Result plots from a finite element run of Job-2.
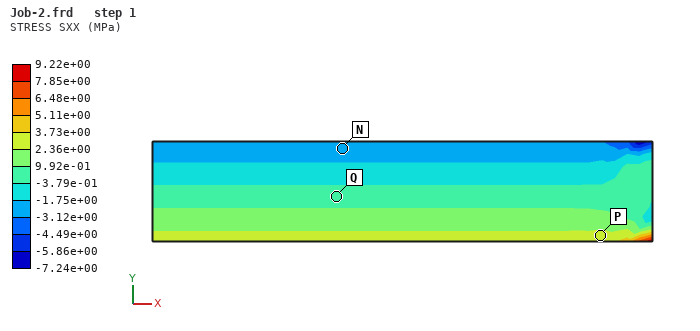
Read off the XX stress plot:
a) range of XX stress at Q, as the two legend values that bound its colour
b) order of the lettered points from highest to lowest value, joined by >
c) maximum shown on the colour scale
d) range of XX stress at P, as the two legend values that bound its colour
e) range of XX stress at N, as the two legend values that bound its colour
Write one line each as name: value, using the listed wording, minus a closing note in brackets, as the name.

range of XX stress at Q, as the two legend values that bound its colour: -3.79e-01 to 9.92e-01 MPa
order of the lettered points from highest to lowest value, joined by >: P > Q > N
maximum shown on the colour scale: 9.22e+00 MPa
range of XX stress at P, as the two legend values that bound its colour: 2.36e+00 to 3.73e+00 MPa
range of XX stress at N, as the two legend values that bound its colour: -3.12e+00 to -1.75e+00 MPa
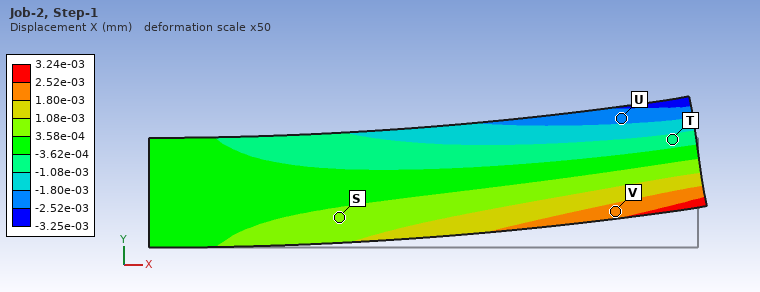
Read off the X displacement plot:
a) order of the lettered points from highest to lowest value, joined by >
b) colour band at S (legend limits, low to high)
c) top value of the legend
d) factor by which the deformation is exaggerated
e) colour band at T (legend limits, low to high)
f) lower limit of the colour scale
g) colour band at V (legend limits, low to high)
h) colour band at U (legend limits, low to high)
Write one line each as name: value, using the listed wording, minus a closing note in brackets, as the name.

order of the lettered points from highest to lowest value, joined by >: V > S > T > U
colour band at S: 3.58e-04 to 1.08e-03 mm
top value of the legend: 3.24e-03 mm
factor by which the deformation is exaggerated: 50
colour band at T: -1.08e-03 to -3.62e-04 mm
lower limit of the colour scale: -3.25e-03 mm
colour band at V: 1.80e-03 to 2.52e-03 mm
colour band at U: -2.52e-03 to -1.80e-03 mm
